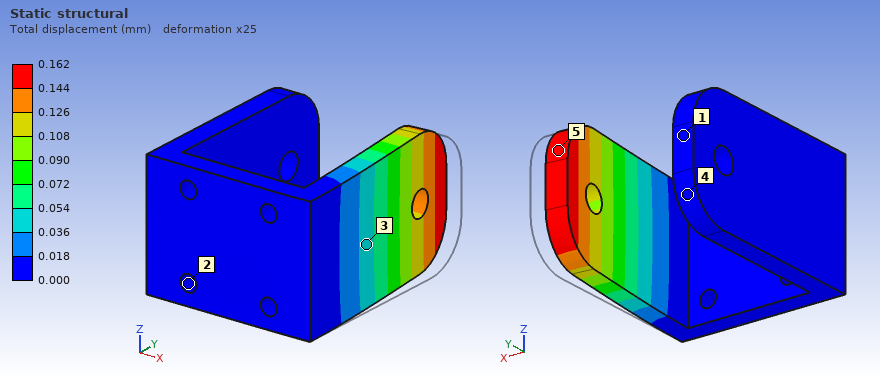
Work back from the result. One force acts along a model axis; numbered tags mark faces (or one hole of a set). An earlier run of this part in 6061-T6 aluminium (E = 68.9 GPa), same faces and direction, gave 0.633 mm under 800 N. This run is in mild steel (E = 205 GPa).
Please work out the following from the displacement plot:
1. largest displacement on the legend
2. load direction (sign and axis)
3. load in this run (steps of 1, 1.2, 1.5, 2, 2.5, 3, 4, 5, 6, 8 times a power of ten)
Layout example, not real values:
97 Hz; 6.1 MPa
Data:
0.162 mm; -X; 600 N
